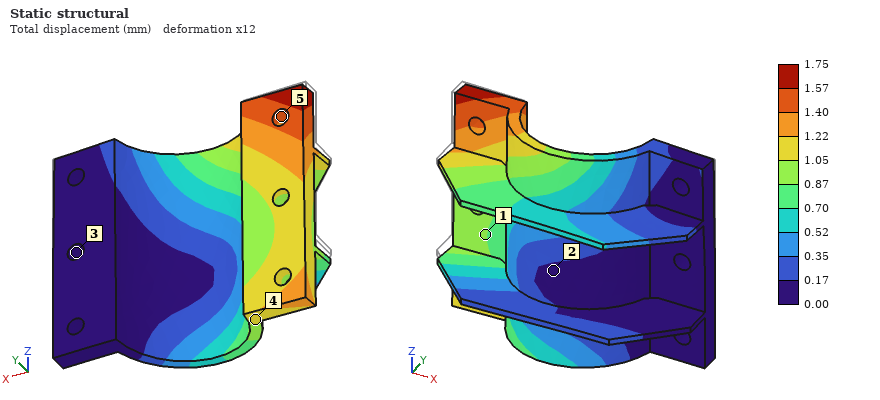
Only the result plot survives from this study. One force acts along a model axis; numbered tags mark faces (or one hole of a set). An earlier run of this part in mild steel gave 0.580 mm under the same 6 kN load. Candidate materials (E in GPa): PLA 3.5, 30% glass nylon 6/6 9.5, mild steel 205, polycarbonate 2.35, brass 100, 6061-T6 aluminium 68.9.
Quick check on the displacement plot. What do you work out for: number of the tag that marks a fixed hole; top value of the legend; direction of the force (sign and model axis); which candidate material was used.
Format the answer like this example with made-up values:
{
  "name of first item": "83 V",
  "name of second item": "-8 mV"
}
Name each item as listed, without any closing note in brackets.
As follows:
{
  "number of the tag that marks a fixed hole": "3",
  "top value of the legend": "1.75 mm",
  "direction of the force": "-Z",
  "which candidate material was used": "6061-T6 aluminium"
}
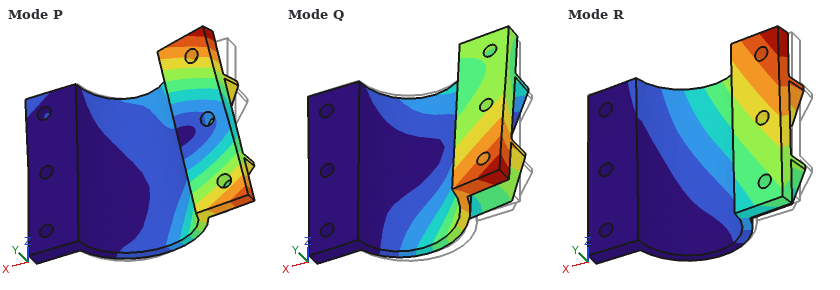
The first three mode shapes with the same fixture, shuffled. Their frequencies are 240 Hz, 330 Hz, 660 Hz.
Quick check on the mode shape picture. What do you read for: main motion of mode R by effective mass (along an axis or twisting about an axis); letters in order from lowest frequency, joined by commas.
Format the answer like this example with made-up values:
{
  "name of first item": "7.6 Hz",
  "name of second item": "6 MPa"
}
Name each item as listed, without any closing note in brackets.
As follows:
{
  "main motion of mode R by effective mass": "along Y",
  "letters in order from lowest frequency, joined by commas": "R, Q, P"
}
